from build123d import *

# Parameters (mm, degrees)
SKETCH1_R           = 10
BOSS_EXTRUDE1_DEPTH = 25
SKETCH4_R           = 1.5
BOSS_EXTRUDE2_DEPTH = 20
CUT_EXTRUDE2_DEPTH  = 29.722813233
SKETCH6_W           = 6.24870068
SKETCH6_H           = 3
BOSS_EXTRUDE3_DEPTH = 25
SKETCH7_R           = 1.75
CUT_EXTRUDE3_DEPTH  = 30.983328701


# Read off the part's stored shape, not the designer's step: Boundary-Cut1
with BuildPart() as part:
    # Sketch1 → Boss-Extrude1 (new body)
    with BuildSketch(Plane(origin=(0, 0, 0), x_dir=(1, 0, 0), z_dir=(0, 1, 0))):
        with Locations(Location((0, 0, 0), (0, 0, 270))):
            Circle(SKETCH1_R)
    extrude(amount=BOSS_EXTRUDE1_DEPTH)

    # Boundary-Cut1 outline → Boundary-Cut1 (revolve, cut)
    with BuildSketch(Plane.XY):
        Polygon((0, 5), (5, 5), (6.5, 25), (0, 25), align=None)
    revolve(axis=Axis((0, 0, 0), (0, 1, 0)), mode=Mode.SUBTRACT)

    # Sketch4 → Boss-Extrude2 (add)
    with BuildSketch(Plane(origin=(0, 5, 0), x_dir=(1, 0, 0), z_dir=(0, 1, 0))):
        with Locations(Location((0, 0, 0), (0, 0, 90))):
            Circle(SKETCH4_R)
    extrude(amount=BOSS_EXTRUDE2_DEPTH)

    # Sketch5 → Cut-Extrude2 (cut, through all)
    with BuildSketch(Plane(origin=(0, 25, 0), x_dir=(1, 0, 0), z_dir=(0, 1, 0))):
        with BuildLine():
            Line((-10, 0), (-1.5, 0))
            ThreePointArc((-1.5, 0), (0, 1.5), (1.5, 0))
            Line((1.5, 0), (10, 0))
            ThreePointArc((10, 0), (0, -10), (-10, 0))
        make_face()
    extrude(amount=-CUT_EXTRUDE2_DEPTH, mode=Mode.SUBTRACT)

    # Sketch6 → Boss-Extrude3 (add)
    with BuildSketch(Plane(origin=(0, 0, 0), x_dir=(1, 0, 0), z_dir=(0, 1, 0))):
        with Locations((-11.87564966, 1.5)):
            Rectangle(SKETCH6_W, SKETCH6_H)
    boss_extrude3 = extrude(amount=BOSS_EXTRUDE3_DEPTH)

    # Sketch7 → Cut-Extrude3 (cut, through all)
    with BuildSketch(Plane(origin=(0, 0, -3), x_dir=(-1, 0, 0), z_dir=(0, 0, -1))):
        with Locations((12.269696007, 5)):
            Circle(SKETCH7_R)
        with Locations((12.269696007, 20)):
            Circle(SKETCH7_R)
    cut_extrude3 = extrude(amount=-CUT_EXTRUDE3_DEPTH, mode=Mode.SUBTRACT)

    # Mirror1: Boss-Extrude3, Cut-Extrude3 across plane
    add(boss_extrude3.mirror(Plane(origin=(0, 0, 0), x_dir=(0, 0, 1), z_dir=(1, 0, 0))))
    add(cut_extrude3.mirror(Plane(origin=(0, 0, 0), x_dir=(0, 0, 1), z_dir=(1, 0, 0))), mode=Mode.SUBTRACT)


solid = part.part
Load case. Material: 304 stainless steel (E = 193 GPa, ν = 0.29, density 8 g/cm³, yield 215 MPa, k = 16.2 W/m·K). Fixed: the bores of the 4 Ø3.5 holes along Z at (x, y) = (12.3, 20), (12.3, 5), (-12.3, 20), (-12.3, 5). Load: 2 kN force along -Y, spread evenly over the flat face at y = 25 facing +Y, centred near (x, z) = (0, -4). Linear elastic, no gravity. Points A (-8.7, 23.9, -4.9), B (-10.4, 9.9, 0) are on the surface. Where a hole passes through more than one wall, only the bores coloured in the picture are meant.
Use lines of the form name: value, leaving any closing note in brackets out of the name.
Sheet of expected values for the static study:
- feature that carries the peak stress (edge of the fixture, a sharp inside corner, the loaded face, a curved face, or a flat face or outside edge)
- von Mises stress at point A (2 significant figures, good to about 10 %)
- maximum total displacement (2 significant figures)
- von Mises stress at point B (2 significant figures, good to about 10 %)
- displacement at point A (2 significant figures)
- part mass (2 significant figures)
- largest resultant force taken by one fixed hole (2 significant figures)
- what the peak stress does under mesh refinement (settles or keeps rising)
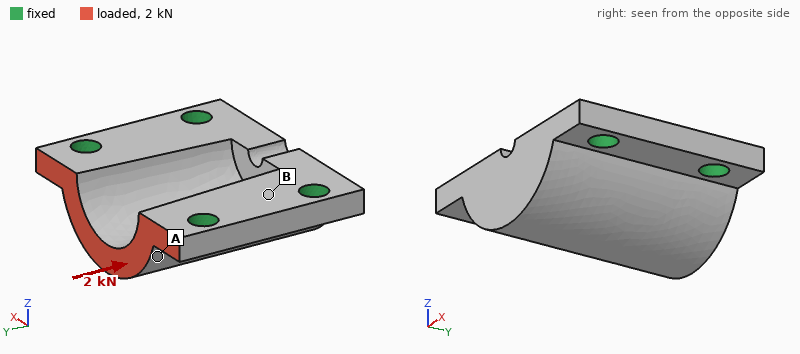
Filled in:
feature that carries the peak stress: edge of the fixture
von Mises stress at point A: 20 MPa
maximum total displacement: 3.4 µm
von Mises stress at point B: 9.6 MPa
displacement at point A: 1.8 µm
part mass: 28 g
largest resultant force taken by one fixed hole: 740 N
what the peak stress does under mesh refinement: keeps rising
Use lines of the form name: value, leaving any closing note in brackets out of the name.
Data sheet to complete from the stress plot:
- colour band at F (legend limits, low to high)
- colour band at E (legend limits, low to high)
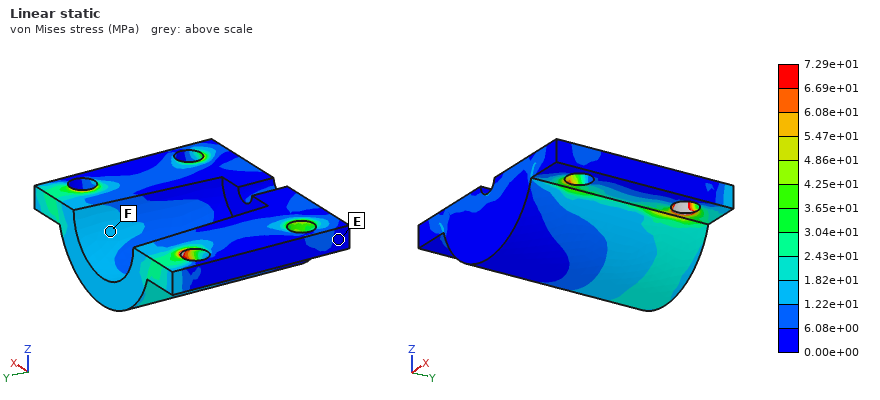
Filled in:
colour band at F: 1.22e+01 to 1.82e+01 MPa
colour band at E: 0.00e+00 to 6.08e+00 MPa
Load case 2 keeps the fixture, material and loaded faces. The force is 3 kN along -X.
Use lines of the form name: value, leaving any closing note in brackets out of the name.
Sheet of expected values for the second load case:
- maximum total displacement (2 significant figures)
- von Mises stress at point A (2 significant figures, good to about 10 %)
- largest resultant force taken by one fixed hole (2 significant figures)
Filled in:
maximum total displacement: 8.2 µm
von Mises stress at point A: 54 MPa
largest resultant force taken by one fixed hole: 1.5 kN
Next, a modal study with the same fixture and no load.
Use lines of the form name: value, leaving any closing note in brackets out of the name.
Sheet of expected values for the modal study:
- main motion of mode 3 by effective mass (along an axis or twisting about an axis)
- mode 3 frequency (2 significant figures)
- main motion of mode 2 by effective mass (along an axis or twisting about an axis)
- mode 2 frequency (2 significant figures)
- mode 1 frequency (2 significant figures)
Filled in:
main motion of mode 3 by effective mass: along X
mode 3 frequency: 47 kHz
main motion of mode 2 by effective mass: along Z
mode 2 frequency: 35 kHz
mode 1 frequency: 29 kHz
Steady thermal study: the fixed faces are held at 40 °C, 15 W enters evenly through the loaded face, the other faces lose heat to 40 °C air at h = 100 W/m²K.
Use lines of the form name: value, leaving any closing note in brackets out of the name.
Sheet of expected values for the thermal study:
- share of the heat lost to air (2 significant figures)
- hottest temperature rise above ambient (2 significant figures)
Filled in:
share of the heat lost to air: 21 %
hottest temperature rise above ambient: 72 K
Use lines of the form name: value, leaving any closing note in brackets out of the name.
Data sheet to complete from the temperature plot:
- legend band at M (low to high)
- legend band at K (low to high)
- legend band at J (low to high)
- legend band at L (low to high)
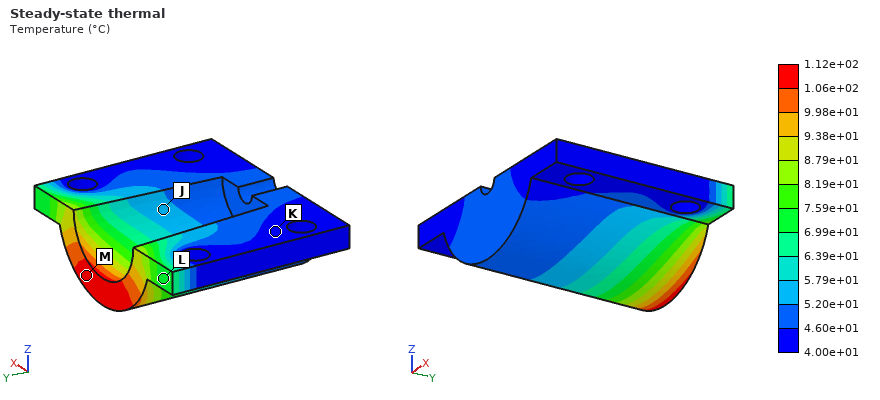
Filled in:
legend band at M: 1.06e+02 to 1.12e+02 °C
legend band at K: 4.00e+01 to 4.60e+01 °C
legend band at J: 5.20e+01 to 5.79e+01 °C
legend band at L: 6.99e+01 to 7.59e+01 °C
